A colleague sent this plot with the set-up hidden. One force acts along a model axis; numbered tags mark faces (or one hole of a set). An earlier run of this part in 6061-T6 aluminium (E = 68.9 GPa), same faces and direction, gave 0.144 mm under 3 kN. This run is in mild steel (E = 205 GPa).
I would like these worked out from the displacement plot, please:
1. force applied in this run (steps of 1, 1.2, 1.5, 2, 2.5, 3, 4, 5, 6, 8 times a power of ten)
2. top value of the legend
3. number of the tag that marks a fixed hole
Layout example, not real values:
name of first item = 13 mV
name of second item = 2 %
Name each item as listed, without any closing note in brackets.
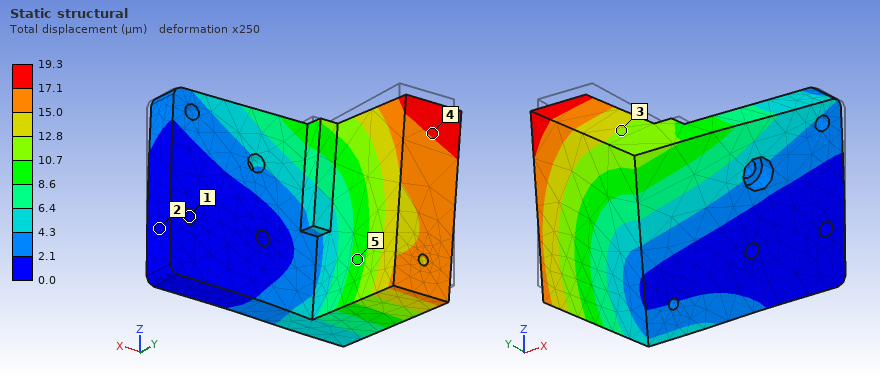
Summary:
force applied in this run = 1.2 kN
top value of the legend = 19.3 µm
number of the tag that marks a fixed hole = 1
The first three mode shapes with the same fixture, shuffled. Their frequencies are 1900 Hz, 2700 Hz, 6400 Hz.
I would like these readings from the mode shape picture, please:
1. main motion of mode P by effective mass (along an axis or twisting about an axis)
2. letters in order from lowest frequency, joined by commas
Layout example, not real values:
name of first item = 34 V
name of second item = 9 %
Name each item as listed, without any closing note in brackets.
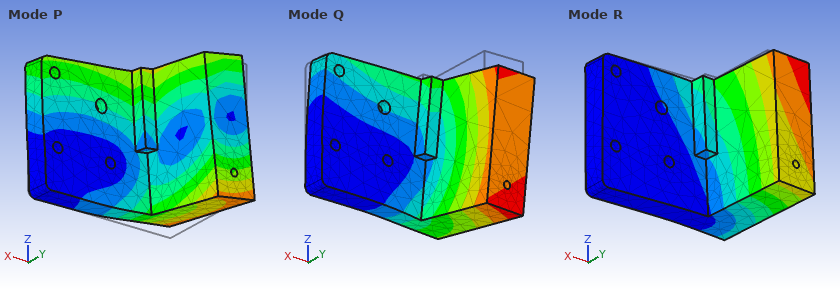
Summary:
main motion of mode P by effective mass = along Z
letters in order from lowest frequency, joined by commas = R, Q, P
